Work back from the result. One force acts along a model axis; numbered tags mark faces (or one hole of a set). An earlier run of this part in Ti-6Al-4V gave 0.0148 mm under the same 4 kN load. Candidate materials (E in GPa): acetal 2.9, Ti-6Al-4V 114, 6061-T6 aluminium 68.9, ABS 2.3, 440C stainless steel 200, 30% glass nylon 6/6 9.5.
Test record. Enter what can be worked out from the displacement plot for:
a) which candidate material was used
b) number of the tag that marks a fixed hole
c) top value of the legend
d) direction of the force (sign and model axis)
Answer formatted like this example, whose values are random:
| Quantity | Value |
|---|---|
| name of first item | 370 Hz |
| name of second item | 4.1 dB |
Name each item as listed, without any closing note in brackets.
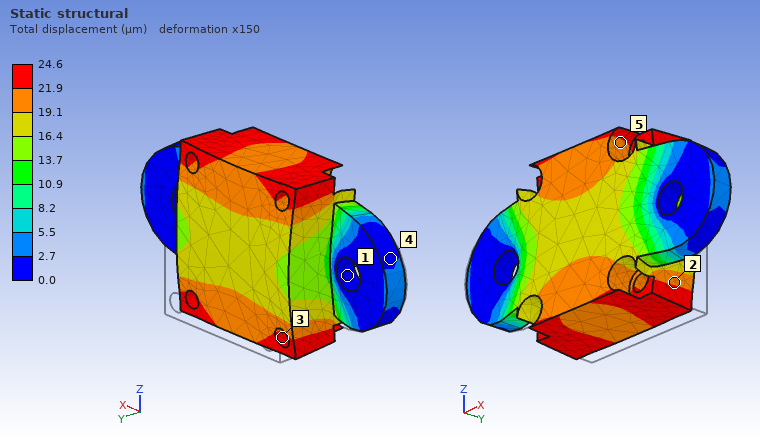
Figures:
| Quantity | Value |
|---|---|
| which candidate material was used | 6061-T6 aluminium |
| number of the tag that marks a fixed hole | 1 |
| top value of the legend | 24.6 µm |
| direction of the force | -Y |
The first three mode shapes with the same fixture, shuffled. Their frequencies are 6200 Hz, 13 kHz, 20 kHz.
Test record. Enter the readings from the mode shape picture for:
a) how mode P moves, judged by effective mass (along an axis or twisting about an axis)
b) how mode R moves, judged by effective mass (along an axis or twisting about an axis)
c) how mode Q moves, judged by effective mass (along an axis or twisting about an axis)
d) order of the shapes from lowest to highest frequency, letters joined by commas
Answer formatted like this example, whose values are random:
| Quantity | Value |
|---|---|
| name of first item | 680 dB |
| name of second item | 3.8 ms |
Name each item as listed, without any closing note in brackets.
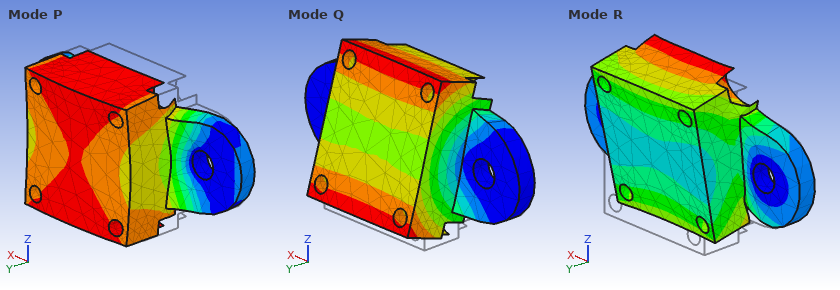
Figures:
| Quantity | Value |
|---|---|
| how mode P moves, judged by effective mass | along Y |
| how mode R moves, judged by effective mass | along Z |
| how mode Q moves, judged by effective mass | along Z |
| order of the shapes from lowest to highest frequency, letters joined by commas | Q, P, R |
